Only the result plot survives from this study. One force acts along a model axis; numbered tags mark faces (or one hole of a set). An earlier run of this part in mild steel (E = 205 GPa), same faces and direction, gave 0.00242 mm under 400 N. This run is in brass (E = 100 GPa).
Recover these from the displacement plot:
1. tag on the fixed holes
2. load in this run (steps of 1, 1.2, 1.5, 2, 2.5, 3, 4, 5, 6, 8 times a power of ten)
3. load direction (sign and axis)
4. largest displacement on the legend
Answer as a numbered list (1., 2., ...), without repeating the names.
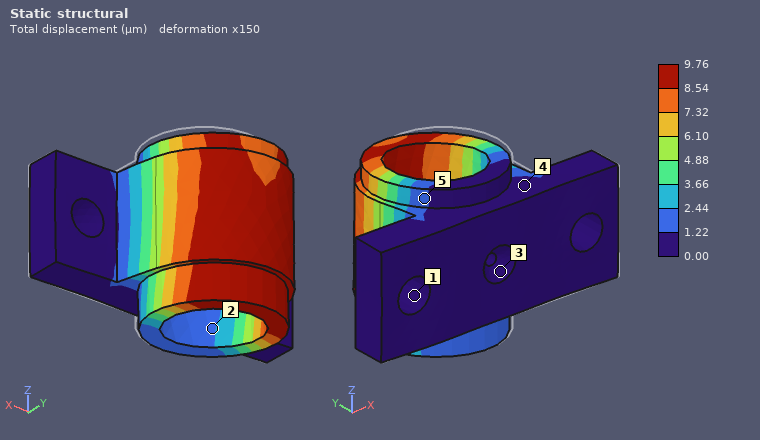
1. 1
2. 800 N
3. -X
4. 9.76 µm
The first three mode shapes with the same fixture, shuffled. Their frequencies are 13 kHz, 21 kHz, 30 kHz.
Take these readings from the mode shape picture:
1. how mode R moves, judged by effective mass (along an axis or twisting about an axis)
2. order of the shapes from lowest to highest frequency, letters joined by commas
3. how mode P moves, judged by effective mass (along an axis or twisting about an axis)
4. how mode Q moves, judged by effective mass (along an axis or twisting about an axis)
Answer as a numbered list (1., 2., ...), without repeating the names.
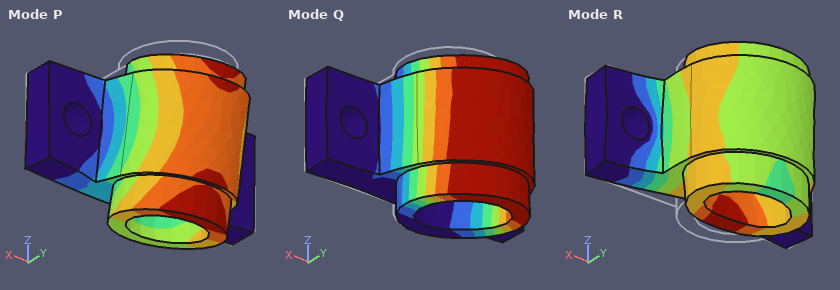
1. along Y
2. P, Q, R
3. along Z
4. along X
